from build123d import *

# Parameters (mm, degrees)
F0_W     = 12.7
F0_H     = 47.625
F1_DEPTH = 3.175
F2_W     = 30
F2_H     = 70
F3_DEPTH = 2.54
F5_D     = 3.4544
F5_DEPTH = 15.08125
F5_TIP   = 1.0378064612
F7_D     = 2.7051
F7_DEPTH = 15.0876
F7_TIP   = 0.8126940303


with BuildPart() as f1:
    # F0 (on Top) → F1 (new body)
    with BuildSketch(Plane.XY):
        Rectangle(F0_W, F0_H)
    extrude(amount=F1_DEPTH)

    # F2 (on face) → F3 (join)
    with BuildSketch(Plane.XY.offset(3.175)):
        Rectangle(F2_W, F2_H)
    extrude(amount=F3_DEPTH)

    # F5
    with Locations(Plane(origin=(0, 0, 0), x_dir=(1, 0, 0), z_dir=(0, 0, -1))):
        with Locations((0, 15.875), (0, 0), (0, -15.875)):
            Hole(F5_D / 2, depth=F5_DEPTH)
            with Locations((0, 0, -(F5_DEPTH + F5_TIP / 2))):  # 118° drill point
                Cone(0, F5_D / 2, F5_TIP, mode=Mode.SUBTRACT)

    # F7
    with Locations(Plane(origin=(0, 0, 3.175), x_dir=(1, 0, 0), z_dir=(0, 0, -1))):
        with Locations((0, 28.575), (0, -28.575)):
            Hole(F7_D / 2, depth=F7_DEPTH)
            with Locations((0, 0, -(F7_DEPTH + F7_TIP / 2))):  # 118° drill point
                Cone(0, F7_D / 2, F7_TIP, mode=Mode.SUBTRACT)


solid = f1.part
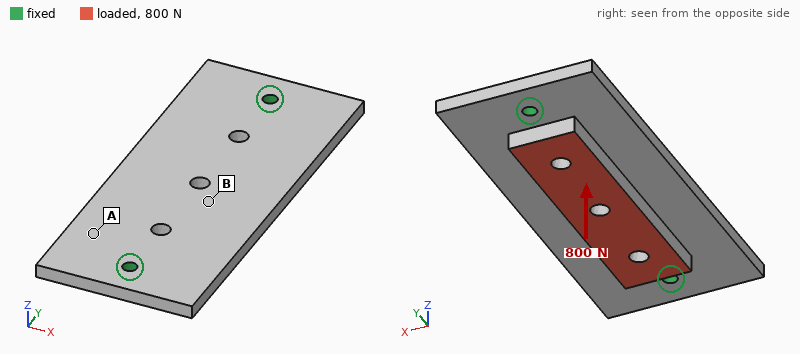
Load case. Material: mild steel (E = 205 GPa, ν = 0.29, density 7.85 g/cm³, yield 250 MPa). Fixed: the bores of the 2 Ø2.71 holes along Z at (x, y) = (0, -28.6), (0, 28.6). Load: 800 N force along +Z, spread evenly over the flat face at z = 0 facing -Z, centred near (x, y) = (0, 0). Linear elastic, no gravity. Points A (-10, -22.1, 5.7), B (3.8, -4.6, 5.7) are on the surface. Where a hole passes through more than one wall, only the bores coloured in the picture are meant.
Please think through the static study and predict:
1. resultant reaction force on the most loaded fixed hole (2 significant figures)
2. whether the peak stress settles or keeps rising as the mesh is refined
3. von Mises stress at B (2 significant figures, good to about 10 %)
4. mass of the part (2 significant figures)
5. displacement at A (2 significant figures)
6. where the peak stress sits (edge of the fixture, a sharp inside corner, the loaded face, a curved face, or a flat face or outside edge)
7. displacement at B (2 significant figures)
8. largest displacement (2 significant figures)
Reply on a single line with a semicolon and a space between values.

660 N; keeps rising; 30 MPa; 55 g; 8.1 µm; edge of the fixture; 23 µm; 25 µm
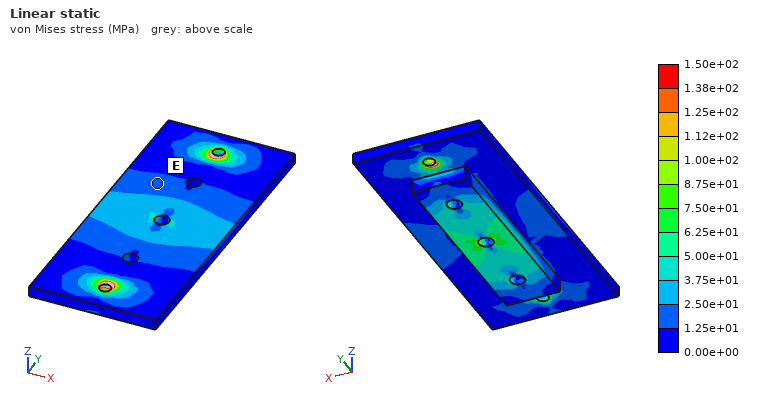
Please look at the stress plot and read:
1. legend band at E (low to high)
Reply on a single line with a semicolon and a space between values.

1.25e+01 to 2.50e+01 MPa
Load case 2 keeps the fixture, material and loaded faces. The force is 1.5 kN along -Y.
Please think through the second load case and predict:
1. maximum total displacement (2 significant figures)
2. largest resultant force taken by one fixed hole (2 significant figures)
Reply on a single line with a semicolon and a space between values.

1.6 µm; 760 N
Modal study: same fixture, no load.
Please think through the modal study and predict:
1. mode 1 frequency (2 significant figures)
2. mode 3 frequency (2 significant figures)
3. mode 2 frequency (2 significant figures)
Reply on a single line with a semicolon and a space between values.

4700 Hz; 9900 Hz; 4900 Hz
